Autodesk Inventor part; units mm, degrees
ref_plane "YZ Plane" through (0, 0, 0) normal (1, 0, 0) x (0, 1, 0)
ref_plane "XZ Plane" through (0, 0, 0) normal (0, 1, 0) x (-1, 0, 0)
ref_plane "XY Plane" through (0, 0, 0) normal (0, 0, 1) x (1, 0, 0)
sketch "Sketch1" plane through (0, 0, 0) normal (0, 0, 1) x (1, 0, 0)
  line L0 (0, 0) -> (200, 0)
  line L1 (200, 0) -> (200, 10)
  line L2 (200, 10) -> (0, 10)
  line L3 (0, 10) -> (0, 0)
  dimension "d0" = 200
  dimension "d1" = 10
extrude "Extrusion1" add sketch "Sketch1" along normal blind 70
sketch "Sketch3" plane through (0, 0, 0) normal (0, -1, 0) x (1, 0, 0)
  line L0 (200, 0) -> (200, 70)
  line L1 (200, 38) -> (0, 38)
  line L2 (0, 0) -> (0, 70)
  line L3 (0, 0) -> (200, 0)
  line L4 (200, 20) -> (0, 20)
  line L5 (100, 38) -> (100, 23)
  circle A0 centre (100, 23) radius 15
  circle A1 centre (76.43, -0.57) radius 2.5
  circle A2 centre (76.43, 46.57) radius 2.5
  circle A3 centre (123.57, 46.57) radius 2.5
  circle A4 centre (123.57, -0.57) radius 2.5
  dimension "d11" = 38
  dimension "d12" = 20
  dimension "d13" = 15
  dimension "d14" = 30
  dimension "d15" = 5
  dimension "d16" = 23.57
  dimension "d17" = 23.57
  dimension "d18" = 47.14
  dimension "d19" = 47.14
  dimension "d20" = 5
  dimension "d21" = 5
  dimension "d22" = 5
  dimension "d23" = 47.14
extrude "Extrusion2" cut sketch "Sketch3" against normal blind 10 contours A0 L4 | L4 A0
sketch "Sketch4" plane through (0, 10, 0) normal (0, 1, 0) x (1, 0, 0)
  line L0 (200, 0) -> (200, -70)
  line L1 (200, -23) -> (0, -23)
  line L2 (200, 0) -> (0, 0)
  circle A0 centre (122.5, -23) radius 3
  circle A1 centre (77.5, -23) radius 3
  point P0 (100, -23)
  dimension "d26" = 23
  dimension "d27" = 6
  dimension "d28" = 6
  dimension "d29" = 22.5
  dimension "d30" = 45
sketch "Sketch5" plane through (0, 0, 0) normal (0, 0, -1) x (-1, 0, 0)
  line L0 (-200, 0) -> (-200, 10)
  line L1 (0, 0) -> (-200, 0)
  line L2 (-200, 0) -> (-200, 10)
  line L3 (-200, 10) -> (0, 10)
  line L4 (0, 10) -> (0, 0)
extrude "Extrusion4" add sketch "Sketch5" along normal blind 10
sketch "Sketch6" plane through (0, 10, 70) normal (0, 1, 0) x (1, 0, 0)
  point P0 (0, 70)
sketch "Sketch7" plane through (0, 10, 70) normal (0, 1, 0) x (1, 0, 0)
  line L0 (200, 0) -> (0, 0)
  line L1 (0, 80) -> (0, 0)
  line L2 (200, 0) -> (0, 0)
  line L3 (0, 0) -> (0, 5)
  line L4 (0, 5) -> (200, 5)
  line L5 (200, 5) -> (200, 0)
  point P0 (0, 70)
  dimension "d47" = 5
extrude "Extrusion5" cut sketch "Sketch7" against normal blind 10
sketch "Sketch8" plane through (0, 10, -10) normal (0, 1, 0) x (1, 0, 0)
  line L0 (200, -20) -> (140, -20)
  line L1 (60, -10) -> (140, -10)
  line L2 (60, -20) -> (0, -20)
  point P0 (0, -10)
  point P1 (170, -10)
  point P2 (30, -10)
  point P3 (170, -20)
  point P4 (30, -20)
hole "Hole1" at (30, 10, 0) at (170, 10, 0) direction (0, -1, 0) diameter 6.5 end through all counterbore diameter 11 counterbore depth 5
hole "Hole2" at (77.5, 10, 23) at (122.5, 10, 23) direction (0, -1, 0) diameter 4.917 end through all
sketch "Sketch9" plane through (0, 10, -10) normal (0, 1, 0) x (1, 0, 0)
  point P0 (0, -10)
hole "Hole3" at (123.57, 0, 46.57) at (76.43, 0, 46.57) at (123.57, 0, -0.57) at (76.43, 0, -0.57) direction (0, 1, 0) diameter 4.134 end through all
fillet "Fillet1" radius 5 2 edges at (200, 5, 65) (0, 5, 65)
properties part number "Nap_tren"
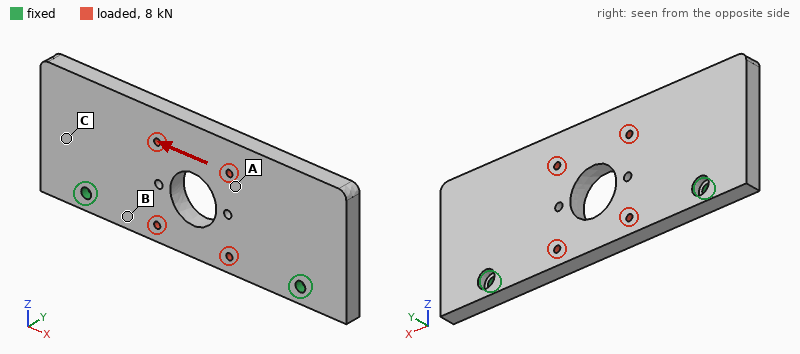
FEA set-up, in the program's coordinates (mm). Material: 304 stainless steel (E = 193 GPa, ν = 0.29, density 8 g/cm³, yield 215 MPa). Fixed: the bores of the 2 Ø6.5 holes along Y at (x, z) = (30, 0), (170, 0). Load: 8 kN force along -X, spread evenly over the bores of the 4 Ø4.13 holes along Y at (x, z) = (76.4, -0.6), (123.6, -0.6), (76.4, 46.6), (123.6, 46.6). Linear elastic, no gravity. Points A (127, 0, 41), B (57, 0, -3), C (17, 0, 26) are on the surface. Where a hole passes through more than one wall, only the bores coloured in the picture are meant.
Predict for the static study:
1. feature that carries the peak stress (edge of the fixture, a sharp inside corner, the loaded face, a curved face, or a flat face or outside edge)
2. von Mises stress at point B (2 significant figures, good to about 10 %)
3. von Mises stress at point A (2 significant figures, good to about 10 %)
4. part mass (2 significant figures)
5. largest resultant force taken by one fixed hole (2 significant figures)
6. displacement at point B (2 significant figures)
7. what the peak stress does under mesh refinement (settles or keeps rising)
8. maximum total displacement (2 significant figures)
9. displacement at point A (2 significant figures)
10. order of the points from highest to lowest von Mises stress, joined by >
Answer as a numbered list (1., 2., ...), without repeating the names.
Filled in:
1. edge of the fixture
2. 18 MPa
3. 11 MPa
4. 1.1 kg
5. 4.2 kN
6. 3.6 µm
7. keeps rising
8. 8.0 µm
9. 6.5 µm
10. B > A > C
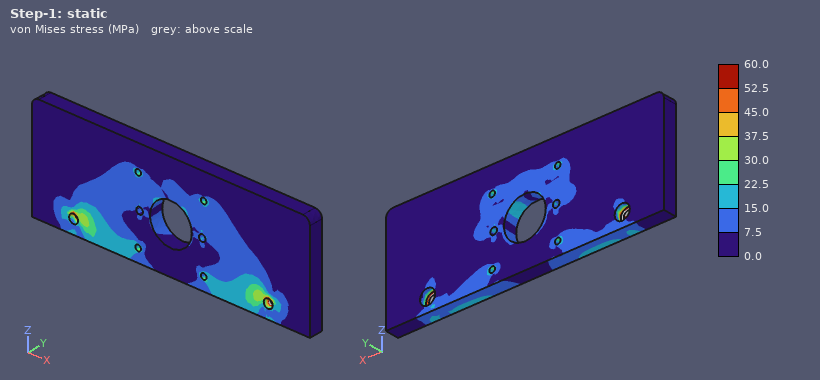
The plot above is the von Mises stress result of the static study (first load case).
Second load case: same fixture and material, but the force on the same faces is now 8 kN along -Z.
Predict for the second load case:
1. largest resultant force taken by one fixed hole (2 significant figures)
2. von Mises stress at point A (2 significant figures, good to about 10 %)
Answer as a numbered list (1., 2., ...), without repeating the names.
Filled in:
1. 4.5 kN
2. 15 MPa
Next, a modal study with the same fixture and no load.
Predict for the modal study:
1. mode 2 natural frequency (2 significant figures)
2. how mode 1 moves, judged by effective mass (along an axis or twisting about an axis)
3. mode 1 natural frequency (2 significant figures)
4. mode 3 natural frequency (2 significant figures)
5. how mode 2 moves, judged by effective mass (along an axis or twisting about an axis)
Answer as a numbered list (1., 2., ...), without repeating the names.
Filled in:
1. 1500 Hz
2. along Y
3. 810 Hz
4. 1700 Hz
5. twisting about Z
